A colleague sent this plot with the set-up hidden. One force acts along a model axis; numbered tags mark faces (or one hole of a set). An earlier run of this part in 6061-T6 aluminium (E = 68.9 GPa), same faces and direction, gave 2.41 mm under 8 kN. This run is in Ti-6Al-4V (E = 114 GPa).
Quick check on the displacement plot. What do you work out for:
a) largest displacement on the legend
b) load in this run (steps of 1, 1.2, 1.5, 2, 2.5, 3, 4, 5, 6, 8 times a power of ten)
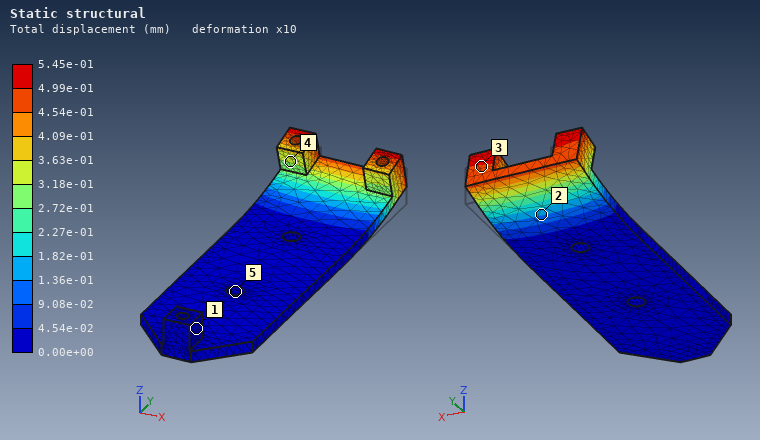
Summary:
5.45e-01 mm
3 kN
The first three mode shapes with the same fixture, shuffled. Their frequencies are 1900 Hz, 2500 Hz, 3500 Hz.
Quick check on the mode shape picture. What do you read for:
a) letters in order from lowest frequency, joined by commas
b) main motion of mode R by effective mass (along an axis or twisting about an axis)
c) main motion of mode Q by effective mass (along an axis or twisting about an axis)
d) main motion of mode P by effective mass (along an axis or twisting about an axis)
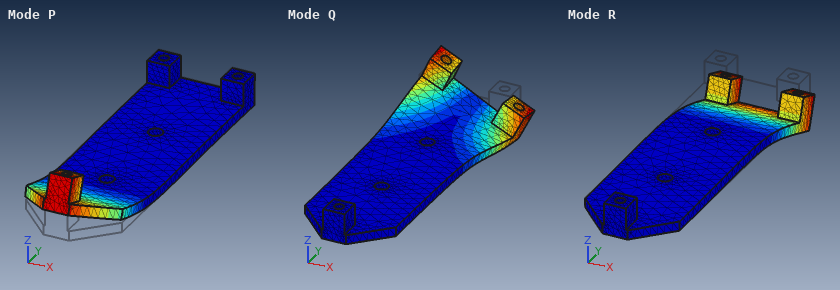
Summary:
R, P, Q
along Z
twisting about Y
along Z
